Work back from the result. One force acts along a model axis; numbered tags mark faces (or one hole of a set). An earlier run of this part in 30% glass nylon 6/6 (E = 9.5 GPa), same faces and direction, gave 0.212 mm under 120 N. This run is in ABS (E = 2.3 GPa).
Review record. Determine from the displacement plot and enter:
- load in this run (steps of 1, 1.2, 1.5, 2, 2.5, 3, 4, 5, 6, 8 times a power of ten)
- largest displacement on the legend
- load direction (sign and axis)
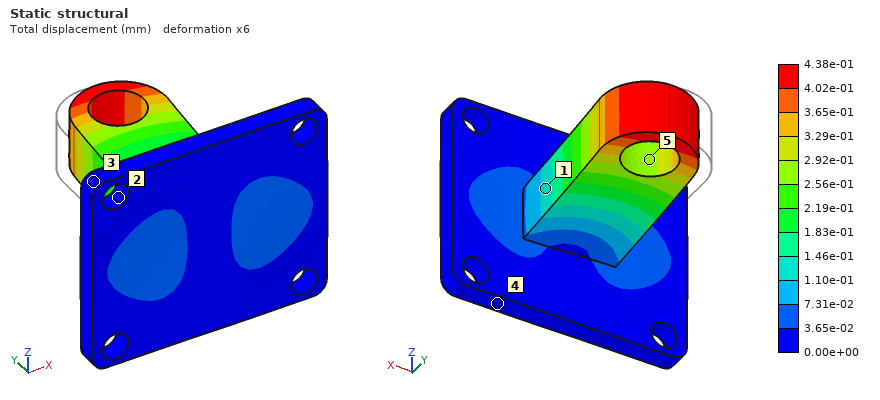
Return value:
60 N
4.38e-01 mm
+X
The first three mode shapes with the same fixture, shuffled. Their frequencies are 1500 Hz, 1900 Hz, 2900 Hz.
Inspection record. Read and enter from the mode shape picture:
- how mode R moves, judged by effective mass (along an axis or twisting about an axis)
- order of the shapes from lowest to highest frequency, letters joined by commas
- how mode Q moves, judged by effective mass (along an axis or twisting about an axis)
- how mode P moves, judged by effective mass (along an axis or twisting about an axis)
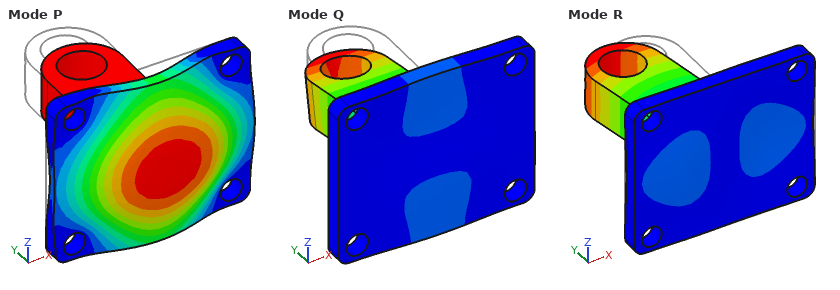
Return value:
along X
Q, R, P
along Z
along Y
